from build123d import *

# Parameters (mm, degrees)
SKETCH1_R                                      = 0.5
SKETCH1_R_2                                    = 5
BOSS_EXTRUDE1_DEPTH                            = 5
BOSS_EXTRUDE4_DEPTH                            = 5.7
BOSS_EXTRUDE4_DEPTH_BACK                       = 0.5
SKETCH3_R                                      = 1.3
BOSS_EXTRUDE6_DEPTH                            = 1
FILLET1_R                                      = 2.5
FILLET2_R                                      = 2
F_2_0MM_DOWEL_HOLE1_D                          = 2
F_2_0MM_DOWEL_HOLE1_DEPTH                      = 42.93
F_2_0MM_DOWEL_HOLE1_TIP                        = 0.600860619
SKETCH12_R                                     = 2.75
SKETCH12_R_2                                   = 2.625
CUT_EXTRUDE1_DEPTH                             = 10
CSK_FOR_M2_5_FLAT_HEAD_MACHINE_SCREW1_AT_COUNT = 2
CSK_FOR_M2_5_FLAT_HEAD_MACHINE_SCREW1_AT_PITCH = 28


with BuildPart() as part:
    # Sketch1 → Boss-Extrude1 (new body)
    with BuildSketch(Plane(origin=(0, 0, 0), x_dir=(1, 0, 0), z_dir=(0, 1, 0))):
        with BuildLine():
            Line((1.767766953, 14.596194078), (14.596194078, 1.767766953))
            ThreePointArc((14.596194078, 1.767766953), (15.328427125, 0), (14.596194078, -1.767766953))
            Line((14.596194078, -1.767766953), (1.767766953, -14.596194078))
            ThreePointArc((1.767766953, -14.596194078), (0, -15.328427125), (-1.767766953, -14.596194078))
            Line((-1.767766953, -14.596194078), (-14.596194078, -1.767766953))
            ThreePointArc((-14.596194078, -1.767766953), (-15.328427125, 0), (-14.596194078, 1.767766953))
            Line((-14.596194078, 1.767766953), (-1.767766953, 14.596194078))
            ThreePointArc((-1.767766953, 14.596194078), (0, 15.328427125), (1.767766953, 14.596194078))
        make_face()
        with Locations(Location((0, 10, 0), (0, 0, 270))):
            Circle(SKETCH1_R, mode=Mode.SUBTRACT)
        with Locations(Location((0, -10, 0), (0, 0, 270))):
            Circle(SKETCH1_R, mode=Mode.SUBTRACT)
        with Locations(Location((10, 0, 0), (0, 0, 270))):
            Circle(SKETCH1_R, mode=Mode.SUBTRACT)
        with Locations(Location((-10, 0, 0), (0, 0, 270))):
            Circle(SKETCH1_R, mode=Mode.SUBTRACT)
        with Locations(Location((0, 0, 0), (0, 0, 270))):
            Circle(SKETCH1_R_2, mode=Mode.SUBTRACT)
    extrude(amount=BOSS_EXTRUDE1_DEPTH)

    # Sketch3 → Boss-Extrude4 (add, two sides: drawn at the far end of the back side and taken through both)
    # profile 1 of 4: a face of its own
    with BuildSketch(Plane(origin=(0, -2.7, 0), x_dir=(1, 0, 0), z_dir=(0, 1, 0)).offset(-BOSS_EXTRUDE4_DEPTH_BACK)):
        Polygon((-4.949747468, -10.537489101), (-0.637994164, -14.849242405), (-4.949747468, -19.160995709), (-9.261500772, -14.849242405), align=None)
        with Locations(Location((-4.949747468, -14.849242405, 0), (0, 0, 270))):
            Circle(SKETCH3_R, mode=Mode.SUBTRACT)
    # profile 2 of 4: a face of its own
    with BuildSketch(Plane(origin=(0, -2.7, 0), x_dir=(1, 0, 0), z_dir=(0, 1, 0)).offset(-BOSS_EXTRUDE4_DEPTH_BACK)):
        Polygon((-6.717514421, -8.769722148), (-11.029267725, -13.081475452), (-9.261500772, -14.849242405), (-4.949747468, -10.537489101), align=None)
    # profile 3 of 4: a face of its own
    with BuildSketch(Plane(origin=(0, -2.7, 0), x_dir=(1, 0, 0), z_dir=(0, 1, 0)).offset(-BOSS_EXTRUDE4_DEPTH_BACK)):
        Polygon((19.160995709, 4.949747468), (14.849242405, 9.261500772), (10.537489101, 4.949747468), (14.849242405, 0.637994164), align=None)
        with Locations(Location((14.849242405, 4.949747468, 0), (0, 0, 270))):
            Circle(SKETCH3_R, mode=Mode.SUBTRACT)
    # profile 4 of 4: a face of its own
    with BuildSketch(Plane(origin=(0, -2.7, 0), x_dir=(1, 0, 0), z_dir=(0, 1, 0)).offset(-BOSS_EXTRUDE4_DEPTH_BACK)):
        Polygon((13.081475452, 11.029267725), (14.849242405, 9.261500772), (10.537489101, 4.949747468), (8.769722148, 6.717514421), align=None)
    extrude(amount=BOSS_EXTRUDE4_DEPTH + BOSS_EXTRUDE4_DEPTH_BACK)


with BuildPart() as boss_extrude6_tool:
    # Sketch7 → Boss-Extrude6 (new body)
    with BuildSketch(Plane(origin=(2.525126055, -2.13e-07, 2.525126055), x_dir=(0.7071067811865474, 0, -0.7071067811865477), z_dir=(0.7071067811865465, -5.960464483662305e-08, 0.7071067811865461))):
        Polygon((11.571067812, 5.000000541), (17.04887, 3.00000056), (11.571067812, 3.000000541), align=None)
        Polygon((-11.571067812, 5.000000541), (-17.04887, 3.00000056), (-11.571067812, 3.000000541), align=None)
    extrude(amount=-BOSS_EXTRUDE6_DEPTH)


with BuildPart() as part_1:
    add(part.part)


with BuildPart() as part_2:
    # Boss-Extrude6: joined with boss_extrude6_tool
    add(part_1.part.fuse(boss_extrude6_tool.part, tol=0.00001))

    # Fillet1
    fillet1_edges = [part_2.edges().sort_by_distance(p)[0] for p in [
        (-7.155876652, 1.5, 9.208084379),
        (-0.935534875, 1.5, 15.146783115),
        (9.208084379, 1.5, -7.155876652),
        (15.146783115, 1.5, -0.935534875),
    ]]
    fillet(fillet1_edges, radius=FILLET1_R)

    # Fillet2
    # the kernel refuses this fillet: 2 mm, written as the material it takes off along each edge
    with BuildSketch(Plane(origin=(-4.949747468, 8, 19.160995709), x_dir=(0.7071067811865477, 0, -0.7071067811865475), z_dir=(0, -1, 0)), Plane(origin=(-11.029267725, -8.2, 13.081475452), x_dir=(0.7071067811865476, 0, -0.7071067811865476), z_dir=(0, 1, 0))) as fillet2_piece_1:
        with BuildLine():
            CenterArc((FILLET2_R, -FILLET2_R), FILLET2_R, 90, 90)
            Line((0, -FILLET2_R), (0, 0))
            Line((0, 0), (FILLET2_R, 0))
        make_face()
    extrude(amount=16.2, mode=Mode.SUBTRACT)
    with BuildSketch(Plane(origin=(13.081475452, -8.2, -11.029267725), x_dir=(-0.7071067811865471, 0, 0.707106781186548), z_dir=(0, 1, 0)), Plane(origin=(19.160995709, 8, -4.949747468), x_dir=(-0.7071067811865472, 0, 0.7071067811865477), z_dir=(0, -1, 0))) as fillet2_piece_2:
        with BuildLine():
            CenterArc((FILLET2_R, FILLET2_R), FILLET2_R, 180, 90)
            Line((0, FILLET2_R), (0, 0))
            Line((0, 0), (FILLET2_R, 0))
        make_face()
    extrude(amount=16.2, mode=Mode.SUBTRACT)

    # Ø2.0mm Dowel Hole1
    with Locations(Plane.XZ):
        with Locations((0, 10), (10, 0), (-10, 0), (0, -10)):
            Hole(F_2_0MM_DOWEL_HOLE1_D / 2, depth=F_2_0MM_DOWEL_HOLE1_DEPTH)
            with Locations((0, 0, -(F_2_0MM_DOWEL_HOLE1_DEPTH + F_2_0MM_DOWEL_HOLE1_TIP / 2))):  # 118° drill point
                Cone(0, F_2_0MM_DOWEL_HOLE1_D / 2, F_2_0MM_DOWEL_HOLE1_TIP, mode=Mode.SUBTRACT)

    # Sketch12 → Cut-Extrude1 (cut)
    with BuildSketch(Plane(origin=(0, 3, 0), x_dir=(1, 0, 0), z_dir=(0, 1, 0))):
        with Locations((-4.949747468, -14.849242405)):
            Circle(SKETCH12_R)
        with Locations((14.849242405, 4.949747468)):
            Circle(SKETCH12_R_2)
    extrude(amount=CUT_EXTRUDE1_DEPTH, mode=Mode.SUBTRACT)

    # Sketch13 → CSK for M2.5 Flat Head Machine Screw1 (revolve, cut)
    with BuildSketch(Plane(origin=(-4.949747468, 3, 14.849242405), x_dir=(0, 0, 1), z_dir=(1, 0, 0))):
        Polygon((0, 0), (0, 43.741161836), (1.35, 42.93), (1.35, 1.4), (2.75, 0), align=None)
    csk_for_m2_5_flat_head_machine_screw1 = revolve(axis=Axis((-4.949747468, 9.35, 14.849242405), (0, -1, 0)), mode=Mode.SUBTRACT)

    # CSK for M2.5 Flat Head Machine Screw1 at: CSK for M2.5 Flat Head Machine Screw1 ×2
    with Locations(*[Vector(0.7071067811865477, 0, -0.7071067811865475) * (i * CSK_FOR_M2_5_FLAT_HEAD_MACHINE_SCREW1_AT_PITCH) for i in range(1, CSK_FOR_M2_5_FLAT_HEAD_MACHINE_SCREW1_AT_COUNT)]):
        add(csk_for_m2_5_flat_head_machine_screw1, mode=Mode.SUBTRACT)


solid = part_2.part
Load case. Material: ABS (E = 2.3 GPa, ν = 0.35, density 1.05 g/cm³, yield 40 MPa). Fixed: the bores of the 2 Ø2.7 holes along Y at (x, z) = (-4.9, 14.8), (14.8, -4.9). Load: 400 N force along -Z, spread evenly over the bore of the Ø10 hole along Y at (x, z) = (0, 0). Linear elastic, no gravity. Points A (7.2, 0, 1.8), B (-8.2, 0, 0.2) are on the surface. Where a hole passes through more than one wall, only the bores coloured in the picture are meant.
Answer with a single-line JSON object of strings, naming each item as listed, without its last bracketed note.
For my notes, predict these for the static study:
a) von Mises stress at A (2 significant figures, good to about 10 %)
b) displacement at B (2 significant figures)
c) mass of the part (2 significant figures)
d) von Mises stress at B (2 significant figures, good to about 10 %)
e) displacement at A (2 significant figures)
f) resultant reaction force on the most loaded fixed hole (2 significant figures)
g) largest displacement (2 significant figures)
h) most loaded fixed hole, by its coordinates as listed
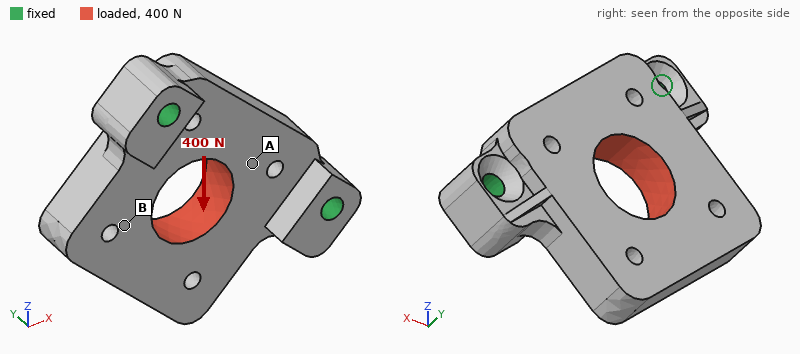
{"von Mises stress at A": "2.5 MPa", "displacement at B": "0.13 mm", "mass of the part": "2.9 g", "von Mises stress at B": "5.3 MPa", "displacement at A": "0.057 mm", "resultant reaction force on the most loaded fixed hole": "260 N", "largest displacement": "0.19 mm", "most loaded fixed hole, by its coordinates as listed": "(-4.9, 14.8)"}
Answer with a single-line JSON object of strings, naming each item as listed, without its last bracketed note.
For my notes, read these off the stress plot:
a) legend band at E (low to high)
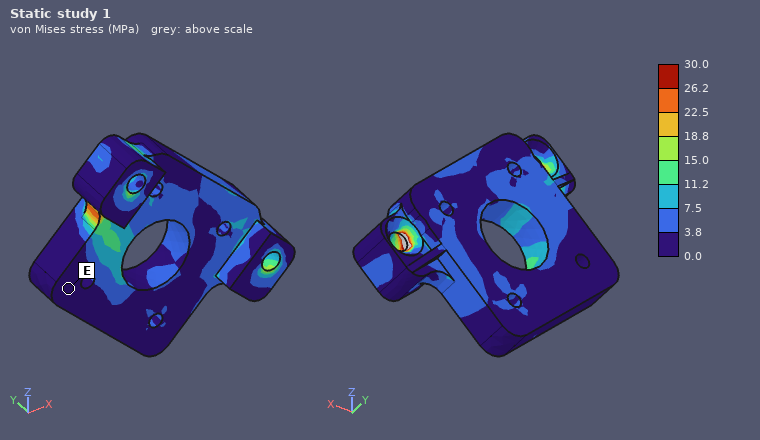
{"legend band at E": "0.0 to 3.8 MPa"}
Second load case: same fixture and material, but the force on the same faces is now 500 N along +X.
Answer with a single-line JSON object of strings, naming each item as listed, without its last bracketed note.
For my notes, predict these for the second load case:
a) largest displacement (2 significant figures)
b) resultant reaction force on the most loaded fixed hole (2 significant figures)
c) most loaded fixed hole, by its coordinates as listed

{"largest displacement": "0.24 mm", "resultant reaction force on the most loaded fixed hole": "330 N", "most loaded fixed hole, by its coordinates as listed": "(14.8, -4.9)"}
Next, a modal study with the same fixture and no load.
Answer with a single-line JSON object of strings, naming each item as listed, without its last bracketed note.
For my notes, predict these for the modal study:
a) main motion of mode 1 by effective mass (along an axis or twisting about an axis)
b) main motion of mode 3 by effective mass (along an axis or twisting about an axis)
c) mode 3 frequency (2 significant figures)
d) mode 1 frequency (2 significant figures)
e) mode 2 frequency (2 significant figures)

{"main motion of mode 1 by effective mass": "along Y", "main motion of mode 3 by effective mass": "along Y", "mode 3 frequency": "7600 Hz", "mode 1 frequency": "2300 Hz", "mode 2 frequency": "5600 Hz"}
